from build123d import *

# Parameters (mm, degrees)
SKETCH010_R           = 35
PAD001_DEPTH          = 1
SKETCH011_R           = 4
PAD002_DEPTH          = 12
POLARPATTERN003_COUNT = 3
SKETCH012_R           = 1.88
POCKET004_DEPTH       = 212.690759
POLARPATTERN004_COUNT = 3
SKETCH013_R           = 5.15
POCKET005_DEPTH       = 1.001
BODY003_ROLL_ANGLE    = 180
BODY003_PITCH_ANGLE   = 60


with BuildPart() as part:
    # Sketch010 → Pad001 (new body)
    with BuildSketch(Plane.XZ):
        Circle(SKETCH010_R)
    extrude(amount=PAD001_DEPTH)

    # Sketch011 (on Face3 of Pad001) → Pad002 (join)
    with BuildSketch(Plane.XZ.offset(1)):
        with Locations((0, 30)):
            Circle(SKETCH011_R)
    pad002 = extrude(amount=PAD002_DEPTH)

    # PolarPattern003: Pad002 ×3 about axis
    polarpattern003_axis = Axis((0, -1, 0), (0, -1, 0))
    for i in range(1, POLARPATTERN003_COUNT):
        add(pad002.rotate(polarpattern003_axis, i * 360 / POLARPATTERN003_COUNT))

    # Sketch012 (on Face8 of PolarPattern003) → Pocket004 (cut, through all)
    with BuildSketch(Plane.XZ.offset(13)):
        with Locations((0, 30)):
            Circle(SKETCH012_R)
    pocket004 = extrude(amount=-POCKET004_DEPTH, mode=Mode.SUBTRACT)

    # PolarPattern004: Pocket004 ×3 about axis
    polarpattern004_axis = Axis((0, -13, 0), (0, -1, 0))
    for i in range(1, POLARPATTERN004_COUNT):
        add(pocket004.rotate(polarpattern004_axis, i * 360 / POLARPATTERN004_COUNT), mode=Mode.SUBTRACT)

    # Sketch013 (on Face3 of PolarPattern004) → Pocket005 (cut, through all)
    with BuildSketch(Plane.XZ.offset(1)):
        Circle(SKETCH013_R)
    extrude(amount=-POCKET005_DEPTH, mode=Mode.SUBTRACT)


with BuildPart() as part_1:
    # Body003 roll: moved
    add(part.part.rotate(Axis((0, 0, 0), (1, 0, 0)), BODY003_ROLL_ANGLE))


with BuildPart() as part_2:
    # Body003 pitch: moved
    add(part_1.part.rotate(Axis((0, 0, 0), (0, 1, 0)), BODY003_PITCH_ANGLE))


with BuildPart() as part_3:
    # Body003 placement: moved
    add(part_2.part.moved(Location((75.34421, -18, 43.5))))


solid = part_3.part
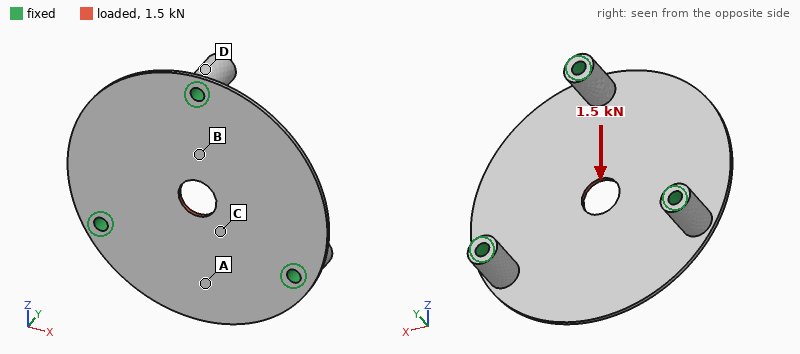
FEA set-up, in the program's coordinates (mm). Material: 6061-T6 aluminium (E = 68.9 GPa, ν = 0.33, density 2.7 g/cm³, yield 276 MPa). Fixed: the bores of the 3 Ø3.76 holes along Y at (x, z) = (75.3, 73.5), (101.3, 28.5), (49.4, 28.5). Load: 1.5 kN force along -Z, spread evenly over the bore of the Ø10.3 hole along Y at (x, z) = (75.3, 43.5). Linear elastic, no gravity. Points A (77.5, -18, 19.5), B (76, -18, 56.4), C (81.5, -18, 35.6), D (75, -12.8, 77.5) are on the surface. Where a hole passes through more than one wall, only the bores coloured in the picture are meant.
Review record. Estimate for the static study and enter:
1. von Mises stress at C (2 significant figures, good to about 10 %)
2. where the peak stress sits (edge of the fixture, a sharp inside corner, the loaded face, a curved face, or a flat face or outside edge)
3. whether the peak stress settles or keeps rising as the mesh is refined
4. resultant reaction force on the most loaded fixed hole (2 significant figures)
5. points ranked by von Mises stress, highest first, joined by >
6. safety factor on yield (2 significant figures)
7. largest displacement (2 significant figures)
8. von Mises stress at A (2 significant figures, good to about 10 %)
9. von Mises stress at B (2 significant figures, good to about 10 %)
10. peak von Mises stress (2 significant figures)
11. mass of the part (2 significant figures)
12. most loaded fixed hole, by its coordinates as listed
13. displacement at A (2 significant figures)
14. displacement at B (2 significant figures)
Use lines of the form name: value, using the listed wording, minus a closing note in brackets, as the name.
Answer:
von Mises stress at C: 30 MPa
where the peak stress sits: the loaded face
whether the peak stress settles or keeps rising as the mesh is refined: settles
resultant reaction force on the most loaded fixed hole: 560 N
points ranked by von Mises stress, highest first, joined by >: B > C > A > D
safety factor on yield: 3.3
largest displacement: 18 µm
von Mises stress at A: 15 MPa
von Mises stress at B: 43 MPa
peak von Mises stress: 83 MPa
mass of the part: 14 g
most loaded fixed hole, by its coordinates as listed: (75.3, 73.5)
displacement at A: 12 µm
displacement at B: 9.6 µm
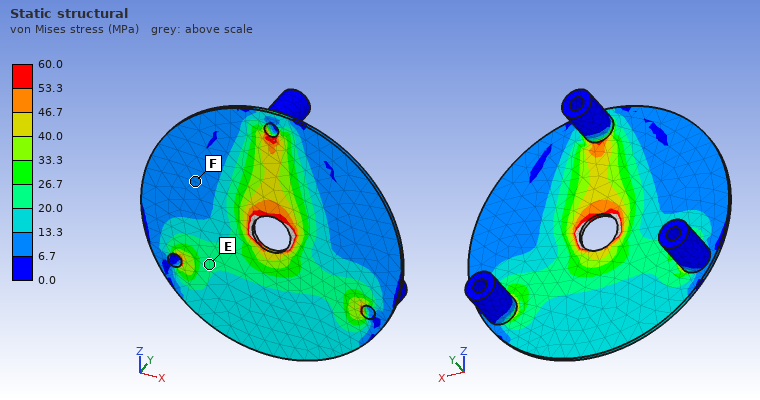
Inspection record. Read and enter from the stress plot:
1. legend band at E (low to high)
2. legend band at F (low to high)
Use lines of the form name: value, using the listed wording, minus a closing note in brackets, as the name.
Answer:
legend band at E: 20.0 to 26.7 MPa
legend band at F: 6.7 to 13.3 MPa
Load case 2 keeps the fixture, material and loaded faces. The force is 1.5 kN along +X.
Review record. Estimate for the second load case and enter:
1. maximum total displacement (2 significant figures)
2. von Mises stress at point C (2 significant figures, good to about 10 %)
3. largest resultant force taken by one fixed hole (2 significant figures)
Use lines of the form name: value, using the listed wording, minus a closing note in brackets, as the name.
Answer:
maximum total displacement: 18 µm
von Mises stress at point C: 36 MPa
largest resultant force taken by one fixed hole: 530 N
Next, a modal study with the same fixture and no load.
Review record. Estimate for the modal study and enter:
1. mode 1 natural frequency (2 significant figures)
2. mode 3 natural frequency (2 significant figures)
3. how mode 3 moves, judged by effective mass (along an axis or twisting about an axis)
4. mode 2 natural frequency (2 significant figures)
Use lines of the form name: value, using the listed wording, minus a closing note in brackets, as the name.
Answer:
mode 1 natural frequency: 1700 Hz
mode 3 natural frequency: 1800 Hz
how mode 3 moves, judged by effective mass: along Y
mode 2 natural frequency: 1700 Hz
